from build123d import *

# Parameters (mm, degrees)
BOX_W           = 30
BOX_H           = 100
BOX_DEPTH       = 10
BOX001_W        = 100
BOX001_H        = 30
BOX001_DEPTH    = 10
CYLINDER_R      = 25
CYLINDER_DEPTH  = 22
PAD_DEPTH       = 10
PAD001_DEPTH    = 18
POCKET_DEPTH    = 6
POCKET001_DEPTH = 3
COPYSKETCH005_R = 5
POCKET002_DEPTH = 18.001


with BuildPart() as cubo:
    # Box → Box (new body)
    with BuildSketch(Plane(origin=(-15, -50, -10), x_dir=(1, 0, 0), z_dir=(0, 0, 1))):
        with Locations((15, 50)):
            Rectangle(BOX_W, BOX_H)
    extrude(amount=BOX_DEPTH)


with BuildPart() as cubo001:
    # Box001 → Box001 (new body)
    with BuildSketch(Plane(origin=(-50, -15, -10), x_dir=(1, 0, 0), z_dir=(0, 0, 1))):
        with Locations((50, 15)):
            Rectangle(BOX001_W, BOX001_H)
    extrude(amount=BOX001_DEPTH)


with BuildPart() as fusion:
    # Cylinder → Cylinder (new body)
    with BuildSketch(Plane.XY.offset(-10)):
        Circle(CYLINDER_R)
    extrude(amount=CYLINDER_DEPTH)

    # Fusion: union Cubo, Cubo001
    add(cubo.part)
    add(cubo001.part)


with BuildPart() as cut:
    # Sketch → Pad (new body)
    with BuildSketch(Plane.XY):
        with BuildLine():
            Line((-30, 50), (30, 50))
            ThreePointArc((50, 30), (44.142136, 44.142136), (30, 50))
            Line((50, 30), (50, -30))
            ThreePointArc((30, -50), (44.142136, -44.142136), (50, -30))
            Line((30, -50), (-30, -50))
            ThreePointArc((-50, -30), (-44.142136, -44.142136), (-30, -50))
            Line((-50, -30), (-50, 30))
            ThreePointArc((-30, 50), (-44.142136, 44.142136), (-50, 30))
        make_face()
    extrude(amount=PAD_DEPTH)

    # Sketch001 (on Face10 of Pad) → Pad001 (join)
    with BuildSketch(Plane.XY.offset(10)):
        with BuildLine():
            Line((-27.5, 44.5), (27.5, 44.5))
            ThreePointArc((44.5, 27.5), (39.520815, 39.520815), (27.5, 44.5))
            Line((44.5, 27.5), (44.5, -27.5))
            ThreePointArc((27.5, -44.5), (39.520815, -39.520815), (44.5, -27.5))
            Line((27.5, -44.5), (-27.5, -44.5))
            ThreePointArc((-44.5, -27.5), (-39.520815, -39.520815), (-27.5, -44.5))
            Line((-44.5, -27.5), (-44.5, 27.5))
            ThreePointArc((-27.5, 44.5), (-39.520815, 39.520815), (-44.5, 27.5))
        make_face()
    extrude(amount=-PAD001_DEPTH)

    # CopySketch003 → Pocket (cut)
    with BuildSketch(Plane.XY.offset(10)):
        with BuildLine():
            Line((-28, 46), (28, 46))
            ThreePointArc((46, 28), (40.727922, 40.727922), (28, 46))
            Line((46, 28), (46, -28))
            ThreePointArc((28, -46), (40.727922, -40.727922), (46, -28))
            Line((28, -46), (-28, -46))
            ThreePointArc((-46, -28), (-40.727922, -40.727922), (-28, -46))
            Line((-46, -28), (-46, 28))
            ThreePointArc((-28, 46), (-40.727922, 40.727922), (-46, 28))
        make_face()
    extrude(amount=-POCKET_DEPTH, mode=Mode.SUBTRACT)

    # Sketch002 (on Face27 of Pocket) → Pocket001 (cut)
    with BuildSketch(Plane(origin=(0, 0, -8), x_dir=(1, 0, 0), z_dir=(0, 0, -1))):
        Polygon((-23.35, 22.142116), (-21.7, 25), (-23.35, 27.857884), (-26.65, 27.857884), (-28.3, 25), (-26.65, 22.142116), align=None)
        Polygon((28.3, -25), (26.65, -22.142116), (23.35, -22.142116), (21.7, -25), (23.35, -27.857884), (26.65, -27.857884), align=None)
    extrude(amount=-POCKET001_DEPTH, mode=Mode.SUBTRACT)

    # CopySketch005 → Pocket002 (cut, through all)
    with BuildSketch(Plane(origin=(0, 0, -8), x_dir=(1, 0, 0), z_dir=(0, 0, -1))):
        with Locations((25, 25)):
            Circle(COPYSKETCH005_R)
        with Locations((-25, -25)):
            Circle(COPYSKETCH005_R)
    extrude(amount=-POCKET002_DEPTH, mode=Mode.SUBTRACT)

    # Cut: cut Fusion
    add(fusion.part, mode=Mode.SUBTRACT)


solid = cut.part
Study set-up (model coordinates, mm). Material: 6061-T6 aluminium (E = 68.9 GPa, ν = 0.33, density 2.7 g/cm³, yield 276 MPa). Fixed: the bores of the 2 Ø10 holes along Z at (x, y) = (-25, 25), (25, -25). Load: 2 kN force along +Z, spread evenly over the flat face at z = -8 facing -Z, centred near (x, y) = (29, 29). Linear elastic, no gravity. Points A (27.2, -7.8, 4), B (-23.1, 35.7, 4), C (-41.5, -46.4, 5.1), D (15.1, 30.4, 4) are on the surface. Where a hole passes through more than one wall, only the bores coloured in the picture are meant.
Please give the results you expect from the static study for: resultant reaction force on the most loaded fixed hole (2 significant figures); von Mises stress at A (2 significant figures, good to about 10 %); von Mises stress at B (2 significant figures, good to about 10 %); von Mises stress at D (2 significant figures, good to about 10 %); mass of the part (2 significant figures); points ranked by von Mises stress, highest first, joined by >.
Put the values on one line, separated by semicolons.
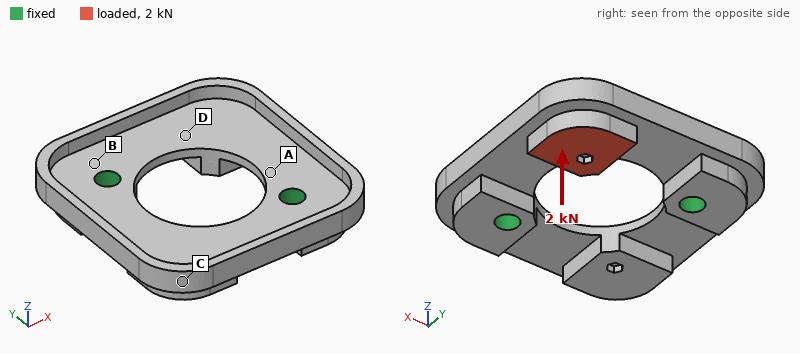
1.1 kN; 110 MPa; 60 MPa; 31 MPa; 170 g; A > B > D > C
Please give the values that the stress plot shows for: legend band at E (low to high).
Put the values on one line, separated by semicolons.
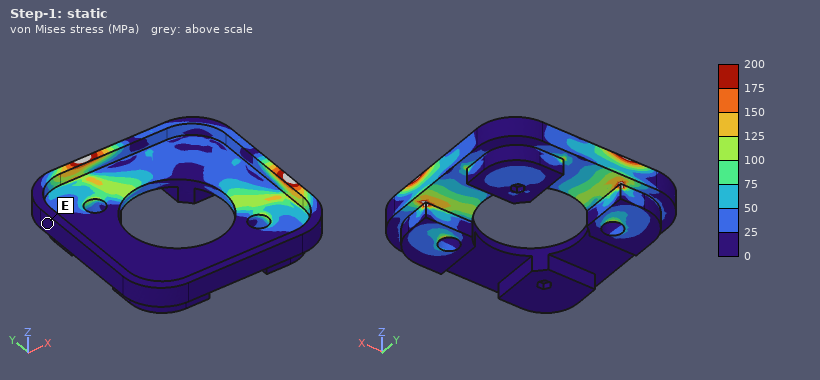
0 to 25 MPa
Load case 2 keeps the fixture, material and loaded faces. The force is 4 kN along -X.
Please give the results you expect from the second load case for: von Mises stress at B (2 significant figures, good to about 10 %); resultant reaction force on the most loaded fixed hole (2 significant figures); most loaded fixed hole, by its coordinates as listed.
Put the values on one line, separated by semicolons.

26 MPa; 3.3 kN; (-25, 25)
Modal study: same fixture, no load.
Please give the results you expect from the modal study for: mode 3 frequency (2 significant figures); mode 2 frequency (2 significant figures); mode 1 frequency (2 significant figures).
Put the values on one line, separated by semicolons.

5200 Hz; 1500 Hz; 1500 Hz
